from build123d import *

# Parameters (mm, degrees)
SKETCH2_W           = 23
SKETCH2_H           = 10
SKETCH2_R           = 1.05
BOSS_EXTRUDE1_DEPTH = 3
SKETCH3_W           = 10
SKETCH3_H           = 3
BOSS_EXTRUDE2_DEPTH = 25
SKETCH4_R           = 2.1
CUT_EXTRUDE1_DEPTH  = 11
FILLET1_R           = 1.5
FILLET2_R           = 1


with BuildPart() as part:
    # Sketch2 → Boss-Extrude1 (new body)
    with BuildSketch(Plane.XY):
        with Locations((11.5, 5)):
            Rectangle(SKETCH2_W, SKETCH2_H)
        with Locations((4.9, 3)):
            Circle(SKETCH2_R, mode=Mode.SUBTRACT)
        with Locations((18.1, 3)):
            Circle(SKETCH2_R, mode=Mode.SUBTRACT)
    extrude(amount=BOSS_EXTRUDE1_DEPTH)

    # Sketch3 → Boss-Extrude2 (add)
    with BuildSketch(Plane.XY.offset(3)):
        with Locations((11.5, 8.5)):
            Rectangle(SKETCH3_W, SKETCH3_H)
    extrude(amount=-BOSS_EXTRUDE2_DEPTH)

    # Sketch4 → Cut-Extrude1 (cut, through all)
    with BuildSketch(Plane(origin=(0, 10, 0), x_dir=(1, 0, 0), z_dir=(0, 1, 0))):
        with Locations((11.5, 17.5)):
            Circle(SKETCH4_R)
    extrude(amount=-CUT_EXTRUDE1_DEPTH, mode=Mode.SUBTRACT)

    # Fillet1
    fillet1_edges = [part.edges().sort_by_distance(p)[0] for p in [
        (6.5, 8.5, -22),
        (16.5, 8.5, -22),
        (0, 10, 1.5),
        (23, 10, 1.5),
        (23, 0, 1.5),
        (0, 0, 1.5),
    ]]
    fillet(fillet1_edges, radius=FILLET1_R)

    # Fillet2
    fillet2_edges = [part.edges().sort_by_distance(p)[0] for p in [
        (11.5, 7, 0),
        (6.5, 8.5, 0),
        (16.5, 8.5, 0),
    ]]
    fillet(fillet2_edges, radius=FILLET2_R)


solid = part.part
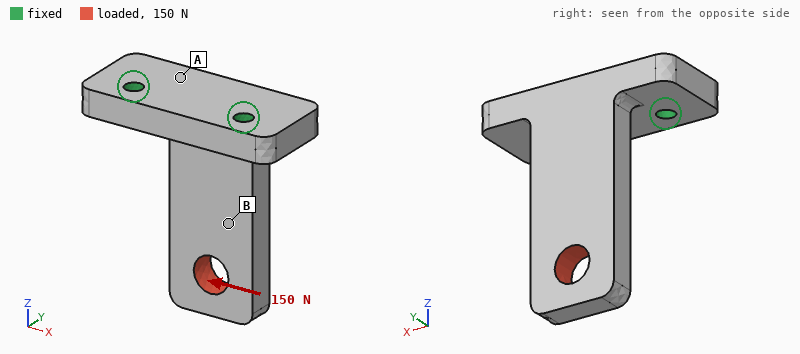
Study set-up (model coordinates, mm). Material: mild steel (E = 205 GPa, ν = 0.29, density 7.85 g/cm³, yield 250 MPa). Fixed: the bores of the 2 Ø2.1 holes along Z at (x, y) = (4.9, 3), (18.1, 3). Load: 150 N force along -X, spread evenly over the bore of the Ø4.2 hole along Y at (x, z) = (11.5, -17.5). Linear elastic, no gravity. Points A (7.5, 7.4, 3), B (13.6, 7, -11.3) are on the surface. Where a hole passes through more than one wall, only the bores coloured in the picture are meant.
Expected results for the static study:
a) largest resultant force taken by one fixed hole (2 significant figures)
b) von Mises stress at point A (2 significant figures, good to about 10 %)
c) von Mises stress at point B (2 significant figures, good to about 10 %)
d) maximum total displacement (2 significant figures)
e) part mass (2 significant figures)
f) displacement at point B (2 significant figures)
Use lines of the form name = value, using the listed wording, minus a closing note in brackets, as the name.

largest resultant force taken by one fixed hole = 240 N
von Mises stress at point A = 36 MPa
von Mises stress at point B = 13 MPa
maximum total displacement = 21 µm
part mass = 10 g
displacement at point B = 9.9 µm
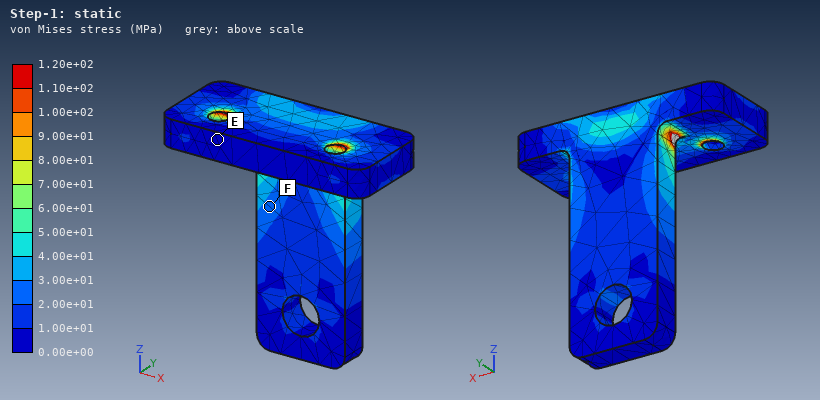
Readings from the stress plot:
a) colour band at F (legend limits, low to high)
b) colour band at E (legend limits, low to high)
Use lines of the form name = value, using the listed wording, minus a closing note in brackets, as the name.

colour band at F = 2.00e+01 to 3.00e+01 MPa
colour band at E = 0.00e+00 to 1.00e+01 MPa
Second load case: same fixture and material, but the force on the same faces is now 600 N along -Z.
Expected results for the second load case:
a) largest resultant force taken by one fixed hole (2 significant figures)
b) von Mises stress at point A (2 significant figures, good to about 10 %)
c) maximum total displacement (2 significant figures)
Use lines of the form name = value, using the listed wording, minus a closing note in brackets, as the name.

largest resultant force taken by one fixed hole = 300 N
von Mises stress at point A = 33 MPa
maximum total displacement = 32 µm
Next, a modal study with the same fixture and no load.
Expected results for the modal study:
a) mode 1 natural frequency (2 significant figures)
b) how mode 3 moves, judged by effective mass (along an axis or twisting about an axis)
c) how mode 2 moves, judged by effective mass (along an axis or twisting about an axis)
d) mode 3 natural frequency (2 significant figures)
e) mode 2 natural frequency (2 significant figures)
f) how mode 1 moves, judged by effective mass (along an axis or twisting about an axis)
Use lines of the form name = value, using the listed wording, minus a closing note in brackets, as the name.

mode 1 natural frequency = 4100 Hz
how mode 3 moves, judged by effective mass = along Z
how mode 2 moves, judged by effective mass = along X
mode 3 natural frequency = 19 kHz
mode 2 natural frequency = 10000 Hz
how mode 1 moves, judged by effective mass = along Y
